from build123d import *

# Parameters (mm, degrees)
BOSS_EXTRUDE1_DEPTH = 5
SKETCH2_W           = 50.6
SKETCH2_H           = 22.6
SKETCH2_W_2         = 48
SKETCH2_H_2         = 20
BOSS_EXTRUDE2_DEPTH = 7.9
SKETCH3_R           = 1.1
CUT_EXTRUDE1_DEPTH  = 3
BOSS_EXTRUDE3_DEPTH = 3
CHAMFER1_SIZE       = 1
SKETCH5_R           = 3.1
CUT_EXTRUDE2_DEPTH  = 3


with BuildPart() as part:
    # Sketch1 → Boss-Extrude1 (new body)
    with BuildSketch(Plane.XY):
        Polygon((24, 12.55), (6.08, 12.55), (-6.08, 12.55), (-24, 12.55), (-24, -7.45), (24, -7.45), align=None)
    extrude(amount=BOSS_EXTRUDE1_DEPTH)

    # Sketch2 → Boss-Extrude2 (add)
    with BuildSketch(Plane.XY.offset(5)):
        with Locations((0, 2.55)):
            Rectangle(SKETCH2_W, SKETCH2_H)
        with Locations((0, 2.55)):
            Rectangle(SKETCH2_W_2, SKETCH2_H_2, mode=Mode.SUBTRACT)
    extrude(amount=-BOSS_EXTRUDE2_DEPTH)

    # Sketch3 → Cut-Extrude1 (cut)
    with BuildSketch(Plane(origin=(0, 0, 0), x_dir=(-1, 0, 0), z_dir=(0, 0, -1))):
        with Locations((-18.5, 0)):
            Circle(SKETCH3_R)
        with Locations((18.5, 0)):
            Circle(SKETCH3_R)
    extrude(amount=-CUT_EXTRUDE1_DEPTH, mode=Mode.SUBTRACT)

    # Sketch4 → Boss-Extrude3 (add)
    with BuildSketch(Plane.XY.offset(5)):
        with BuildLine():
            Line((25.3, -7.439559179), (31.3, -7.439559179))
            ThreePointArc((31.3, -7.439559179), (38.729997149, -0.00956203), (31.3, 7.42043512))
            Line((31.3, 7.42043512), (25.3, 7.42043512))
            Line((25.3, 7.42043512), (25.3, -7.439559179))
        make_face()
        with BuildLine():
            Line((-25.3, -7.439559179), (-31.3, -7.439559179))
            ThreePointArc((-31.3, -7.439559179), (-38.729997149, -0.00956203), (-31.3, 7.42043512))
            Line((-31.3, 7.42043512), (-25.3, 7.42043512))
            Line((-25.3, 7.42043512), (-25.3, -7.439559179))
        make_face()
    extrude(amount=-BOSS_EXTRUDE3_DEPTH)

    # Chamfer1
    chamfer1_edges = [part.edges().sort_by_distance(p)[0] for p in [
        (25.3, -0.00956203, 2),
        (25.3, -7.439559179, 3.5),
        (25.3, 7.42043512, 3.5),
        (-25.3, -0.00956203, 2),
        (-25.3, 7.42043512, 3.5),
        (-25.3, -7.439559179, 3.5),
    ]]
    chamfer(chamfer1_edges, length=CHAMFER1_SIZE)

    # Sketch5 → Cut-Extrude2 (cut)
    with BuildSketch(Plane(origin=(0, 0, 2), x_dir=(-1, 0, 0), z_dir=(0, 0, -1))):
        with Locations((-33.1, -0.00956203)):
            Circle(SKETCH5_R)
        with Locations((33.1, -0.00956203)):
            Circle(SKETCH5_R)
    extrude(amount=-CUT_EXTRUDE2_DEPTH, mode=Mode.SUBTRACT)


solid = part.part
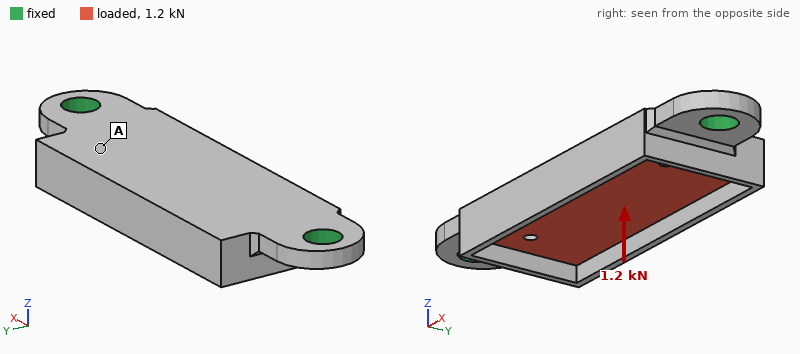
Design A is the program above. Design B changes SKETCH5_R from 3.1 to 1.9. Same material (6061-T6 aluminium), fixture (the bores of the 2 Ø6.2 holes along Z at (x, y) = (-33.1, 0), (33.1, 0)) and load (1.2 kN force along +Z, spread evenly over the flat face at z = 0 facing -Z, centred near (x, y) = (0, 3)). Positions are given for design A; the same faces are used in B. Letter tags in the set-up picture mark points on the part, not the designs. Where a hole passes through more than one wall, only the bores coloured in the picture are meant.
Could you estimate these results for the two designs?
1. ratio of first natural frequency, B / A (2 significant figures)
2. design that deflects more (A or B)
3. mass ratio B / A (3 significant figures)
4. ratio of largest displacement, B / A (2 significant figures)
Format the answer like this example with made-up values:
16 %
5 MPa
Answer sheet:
0.88
B
1.02
1.3
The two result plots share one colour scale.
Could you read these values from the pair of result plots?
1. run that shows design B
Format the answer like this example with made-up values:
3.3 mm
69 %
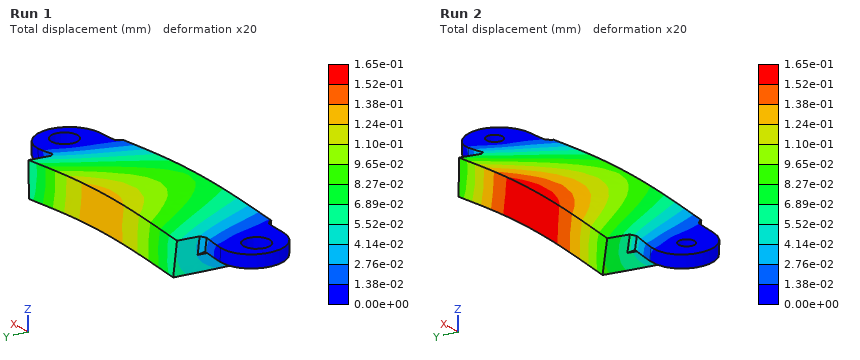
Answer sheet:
Run 2
